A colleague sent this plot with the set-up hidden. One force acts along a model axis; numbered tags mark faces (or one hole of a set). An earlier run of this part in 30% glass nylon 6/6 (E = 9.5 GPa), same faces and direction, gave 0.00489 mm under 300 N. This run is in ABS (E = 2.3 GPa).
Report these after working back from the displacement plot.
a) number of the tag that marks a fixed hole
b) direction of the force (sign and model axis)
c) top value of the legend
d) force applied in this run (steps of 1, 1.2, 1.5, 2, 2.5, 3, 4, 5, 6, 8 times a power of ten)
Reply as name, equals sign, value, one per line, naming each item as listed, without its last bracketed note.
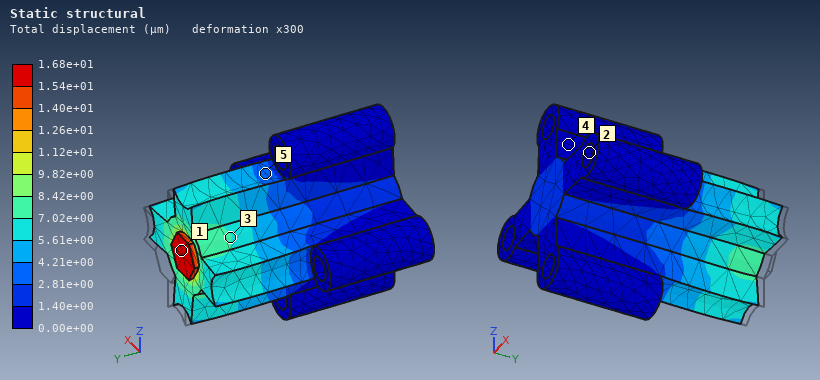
number of the tag that marks a fixed hole = 2
direction of the force = -Y
top value of the legend = 1.68e+01 µm
force applied in this run = 250 N
